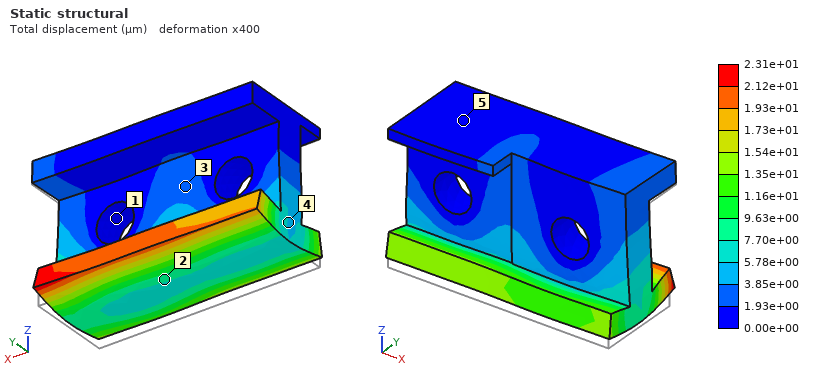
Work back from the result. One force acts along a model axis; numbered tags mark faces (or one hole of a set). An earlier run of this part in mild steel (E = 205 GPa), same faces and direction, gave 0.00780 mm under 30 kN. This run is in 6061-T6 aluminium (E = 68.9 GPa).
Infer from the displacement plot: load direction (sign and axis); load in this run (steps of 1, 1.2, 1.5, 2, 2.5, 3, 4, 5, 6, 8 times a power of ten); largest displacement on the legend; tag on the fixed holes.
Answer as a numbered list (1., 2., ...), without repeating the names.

1. +Z
2. 30 kN
3. 2.31e+01 µm
4. 1
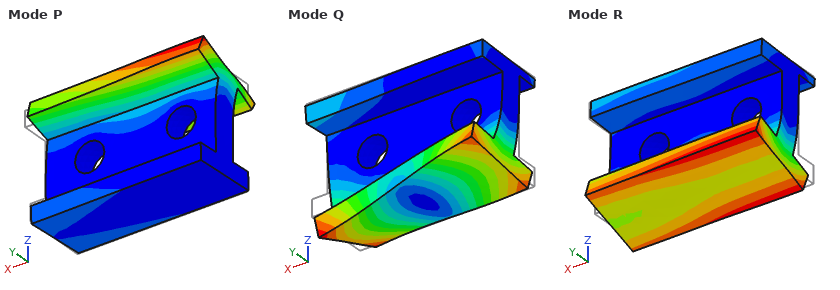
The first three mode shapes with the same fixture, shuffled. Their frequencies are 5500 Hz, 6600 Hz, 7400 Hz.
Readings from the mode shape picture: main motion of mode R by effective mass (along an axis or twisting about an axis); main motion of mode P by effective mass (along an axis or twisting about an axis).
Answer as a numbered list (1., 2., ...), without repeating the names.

1. along Y
2. along Y
